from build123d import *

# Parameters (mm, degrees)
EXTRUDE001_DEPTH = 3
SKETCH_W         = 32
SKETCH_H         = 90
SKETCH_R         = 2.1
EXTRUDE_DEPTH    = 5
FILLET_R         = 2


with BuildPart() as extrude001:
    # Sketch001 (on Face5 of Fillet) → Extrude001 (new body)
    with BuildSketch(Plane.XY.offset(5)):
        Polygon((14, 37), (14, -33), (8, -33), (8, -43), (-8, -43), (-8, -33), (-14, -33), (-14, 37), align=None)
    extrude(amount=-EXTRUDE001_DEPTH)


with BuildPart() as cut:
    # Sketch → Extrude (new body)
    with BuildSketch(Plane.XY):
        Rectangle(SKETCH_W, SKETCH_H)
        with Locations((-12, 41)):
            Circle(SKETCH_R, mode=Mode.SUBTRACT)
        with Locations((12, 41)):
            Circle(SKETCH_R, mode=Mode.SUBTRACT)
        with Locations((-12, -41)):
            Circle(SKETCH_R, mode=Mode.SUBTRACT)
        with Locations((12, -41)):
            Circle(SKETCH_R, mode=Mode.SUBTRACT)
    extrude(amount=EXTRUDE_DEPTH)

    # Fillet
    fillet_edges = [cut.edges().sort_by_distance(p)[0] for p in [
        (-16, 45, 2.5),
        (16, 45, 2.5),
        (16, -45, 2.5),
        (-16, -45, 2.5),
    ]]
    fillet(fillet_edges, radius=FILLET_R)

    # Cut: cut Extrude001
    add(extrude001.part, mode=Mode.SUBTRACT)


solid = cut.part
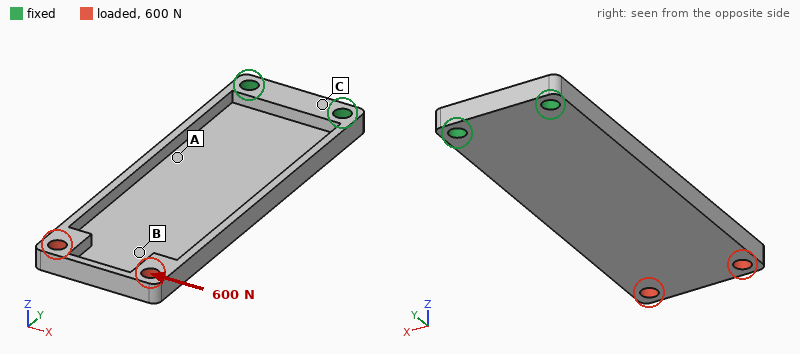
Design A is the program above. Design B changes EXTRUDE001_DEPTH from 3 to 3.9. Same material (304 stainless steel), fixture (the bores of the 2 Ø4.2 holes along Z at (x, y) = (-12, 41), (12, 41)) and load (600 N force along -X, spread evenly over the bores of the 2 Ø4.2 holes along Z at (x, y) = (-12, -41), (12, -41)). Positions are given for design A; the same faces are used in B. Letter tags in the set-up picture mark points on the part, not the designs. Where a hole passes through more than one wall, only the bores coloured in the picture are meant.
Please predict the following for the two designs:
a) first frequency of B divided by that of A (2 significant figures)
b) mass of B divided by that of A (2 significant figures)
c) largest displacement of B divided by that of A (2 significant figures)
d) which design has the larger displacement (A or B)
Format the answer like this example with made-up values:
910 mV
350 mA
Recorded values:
1.1
0.75
2.5
B
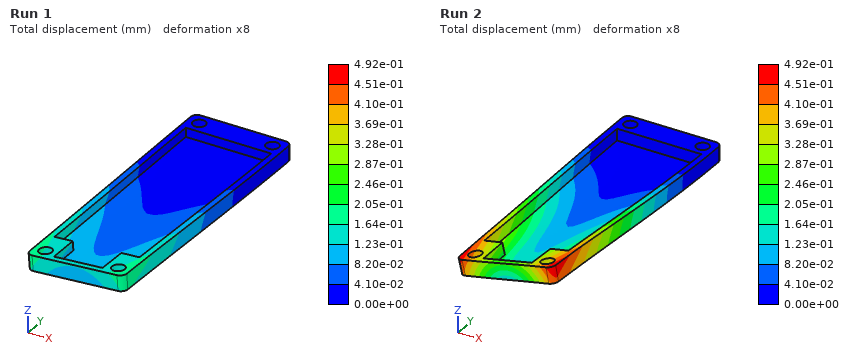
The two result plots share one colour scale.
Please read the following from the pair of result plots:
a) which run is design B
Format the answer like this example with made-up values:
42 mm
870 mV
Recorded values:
Run 2
